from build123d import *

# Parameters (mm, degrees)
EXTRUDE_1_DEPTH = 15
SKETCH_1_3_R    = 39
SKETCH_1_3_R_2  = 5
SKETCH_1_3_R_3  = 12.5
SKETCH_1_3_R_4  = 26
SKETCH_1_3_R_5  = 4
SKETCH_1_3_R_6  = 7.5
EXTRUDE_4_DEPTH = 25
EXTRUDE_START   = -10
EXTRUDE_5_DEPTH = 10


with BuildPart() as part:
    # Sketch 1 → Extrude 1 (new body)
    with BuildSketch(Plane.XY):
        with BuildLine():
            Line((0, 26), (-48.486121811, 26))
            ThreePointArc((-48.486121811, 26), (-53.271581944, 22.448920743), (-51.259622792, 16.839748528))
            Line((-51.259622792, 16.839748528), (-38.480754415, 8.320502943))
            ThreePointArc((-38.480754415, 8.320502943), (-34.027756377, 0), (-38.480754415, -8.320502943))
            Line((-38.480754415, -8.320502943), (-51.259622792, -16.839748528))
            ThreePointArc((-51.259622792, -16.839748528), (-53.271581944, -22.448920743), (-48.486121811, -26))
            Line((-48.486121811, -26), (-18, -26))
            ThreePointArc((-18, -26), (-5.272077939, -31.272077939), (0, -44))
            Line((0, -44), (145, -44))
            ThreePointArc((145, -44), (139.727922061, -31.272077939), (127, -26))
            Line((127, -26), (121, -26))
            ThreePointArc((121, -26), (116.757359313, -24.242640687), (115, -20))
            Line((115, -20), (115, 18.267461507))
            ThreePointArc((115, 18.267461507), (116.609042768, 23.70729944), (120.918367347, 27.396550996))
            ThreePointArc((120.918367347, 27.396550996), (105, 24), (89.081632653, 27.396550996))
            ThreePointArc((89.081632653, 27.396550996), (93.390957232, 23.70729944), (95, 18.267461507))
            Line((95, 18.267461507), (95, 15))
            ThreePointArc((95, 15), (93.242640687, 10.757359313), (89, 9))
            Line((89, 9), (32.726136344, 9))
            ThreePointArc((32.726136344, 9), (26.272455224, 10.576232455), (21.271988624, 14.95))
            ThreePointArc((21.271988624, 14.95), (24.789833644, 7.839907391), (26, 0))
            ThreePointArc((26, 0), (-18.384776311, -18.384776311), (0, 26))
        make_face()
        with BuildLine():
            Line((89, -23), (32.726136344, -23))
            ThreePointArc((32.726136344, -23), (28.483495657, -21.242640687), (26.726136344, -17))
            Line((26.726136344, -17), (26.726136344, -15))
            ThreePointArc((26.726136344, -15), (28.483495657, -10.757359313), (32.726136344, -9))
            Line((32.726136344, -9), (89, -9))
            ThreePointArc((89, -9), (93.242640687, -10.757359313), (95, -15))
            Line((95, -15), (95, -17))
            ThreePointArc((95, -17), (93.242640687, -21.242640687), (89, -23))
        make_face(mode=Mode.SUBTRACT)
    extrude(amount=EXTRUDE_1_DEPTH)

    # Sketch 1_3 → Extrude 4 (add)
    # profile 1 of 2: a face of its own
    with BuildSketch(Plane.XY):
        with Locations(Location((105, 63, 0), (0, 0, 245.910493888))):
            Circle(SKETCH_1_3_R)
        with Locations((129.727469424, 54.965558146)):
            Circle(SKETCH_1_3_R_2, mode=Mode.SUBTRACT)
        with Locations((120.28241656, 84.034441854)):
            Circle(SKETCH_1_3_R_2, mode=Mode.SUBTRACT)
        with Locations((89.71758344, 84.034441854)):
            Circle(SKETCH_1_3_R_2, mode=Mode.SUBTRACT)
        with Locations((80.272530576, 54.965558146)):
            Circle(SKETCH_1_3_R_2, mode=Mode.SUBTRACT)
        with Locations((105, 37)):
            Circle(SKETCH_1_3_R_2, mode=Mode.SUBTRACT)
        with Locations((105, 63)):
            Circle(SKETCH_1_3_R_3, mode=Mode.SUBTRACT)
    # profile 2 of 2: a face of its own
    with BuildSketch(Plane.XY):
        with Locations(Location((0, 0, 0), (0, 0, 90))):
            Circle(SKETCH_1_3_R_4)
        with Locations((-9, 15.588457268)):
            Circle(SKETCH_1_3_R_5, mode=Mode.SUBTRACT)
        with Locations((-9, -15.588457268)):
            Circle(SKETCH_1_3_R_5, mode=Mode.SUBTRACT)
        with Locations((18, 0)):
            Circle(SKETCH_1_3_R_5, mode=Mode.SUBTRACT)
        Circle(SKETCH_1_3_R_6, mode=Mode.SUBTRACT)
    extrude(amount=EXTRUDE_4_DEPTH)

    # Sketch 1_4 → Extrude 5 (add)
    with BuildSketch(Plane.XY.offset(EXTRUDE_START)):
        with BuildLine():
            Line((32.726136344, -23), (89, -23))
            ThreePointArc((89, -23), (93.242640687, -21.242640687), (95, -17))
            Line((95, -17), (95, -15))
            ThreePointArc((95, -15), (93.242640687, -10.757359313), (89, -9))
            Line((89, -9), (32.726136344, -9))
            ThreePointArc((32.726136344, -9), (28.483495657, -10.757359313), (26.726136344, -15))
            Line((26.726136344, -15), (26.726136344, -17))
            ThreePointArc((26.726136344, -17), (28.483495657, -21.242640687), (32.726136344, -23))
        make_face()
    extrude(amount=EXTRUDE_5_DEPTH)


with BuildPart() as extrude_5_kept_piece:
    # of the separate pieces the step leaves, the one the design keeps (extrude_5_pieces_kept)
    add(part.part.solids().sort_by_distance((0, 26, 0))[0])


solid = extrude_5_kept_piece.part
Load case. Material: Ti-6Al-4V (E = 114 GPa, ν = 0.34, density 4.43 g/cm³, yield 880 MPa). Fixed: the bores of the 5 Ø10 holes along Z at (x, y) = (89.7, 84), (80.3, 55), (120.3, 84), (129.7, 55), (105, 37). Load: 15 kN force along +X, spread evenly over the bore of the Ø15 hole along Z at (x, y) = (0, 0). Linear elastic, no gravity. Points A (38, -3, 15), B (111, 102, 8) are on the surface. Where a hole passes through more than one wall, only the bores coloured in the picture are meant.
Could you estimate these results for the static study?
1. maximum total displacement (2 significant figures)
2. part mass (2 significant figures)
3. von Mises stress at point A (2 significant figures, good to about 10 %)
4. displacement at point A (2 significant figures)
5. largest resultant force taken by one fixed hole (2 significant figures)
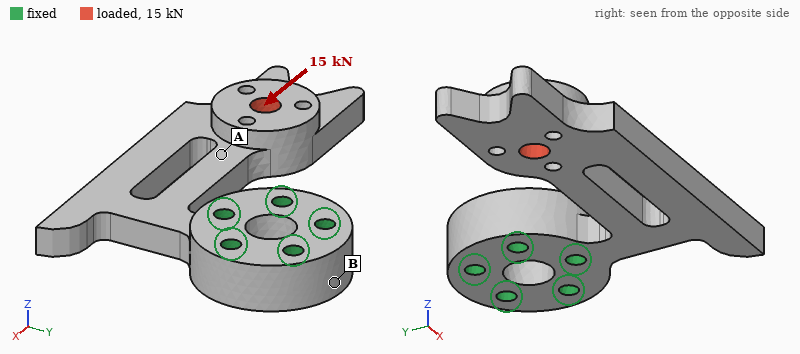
1.5 mm
1.1 kg
100 MPa
0.56 mm
10 kN
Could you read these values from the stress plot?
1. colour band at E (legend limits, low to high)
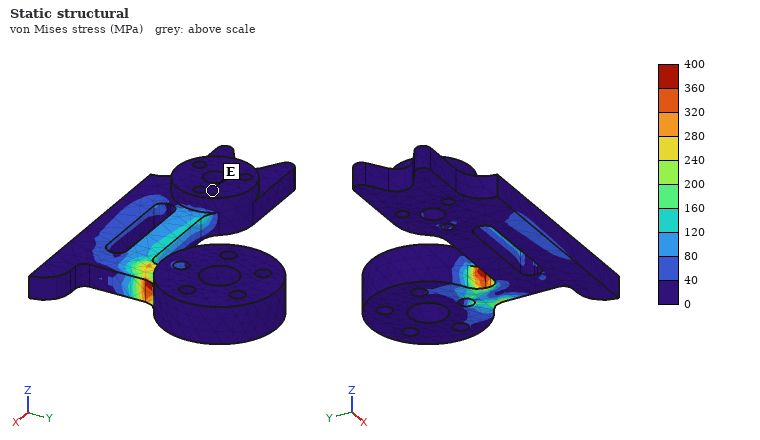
0 to 40 MPa
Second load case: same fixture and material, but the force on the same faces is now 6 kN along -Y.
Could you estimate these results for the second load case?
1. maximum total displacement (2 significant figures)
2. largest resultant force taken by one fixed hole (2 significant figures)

2.9 mm
13 kN
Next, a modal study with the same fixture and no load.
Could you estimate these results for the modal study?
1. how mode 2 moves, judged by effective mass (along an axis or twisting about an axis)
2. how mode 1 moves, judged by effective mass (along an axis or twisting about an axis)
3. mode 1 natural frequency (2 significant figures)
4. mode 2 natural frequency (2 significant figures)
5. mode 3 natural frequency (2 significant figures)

along Y
along Z
270 Hz
410 Hz
910 Hz
